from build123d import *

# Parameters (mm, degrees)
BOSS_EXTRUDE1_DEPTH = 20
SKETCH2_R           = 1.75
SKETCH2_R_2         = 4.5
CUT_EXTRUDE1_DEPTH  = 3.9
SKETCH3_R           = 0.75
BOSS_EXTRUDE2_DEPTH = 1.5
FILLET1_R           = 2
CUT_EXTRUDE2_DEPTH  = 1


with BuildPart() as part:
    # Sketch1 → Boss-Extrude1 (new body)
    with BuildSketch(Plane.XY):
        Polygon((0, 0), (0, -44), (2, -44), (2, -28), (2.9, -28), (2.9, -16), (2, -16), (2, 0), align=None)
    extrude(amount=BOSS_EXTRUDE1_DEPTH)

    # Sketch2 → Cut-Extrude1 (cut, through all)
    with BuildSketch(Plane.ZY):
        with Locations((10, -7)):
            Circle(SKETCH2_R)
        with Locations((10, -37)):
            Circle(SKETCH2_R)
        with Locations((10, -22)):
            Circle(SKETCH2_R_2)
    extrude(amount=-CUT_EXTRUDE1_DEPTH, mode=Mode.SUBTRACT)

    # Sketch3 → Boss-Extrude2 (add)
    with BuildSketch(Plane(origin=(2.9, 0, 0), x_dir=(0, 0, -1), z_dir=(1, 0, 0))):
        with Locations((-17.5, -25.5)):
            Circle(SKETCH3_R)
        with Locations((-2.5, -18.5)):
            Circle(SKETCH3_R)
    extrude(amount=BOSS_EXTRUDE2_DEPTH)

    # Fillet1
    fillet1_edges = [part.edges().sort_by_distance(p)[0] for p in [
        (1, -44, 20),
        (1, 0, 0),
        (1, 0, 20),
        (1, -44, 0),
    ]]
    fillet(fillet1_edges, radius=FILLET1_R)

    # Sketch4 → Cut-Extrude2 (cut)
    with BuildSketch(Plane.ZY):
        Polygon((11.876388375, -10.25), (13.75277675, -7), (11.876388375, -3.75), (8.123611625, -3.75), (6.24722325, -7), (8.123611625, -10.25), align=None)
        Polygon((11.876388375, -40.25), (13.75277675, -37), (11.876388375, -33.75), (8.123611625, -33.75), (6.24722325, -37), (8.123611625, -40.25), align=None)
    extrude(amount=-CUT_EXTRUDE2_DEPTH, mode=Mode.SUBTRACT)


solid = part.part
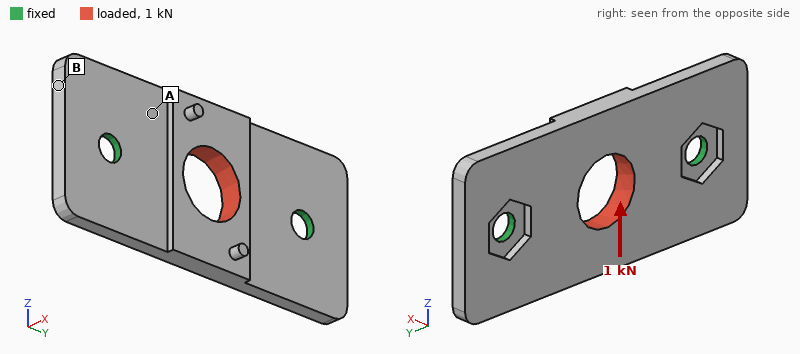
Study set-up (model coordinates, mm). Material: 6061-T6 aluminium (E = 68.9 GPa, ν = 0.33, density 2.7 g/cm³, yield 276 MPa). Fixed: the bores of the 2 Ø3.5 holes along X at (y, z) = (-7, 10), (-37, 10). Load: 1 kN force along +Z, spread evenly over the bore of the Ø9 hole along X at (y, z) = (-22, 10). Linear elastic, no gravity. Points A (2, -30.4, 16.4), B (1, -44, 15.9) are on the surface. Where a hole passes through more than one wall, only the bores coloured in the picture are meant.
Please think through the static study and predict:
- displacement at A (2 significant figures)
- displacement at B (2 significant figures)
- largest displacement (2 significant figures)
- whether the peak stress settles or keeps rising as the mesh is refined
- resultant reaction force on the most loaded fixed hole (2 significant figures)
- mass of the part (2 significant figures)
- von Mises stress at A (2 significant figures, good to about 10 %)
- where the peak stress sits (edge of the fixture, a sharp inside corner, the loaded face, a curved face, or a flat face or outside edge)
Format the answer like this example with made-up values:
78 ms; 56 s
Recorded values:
7.9 µm; 5.1 µm; 15 µm; keeps rising; 500 N; 4.6 g; 33 MPa; edge of the fixture
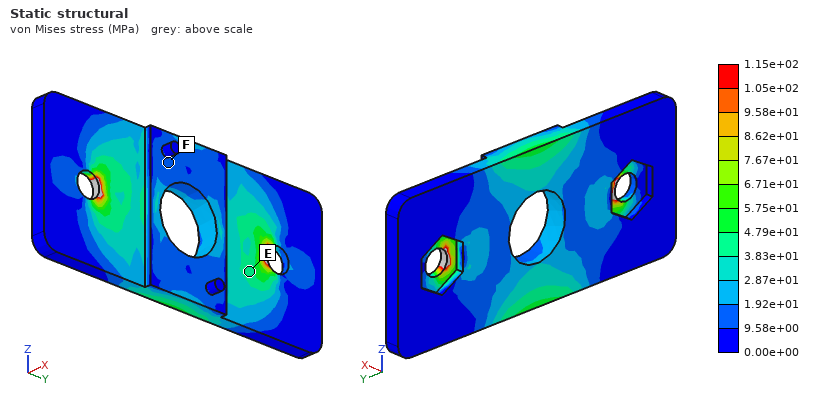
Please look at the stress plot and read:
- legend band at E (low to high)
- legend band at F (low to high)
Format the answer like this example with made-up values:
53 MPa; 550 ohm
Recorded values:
3.83e+01 to 4.79e+01 MPa; 9.58e+00 to 1.92e+01 MPa
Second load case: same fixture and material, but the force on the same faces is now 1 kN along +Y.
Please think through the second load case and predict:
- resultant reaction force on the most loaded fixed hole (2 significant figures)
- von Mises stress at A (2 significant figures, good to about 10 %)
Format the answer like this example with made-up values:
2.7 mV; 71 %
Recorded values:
500 N; 21 MPa
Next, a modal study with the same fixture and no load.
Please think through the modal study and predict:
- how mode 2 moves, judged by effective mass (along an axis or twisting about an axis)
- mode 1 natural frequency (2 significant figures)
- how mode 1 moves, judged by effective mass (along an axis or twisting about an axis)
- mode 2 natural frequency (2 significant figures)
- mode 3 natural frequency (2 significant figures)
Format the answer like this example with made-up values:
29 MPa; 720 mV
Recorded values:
along X; 6500 Hz; twisting about Y; 8200 Hz; 12 kHz
